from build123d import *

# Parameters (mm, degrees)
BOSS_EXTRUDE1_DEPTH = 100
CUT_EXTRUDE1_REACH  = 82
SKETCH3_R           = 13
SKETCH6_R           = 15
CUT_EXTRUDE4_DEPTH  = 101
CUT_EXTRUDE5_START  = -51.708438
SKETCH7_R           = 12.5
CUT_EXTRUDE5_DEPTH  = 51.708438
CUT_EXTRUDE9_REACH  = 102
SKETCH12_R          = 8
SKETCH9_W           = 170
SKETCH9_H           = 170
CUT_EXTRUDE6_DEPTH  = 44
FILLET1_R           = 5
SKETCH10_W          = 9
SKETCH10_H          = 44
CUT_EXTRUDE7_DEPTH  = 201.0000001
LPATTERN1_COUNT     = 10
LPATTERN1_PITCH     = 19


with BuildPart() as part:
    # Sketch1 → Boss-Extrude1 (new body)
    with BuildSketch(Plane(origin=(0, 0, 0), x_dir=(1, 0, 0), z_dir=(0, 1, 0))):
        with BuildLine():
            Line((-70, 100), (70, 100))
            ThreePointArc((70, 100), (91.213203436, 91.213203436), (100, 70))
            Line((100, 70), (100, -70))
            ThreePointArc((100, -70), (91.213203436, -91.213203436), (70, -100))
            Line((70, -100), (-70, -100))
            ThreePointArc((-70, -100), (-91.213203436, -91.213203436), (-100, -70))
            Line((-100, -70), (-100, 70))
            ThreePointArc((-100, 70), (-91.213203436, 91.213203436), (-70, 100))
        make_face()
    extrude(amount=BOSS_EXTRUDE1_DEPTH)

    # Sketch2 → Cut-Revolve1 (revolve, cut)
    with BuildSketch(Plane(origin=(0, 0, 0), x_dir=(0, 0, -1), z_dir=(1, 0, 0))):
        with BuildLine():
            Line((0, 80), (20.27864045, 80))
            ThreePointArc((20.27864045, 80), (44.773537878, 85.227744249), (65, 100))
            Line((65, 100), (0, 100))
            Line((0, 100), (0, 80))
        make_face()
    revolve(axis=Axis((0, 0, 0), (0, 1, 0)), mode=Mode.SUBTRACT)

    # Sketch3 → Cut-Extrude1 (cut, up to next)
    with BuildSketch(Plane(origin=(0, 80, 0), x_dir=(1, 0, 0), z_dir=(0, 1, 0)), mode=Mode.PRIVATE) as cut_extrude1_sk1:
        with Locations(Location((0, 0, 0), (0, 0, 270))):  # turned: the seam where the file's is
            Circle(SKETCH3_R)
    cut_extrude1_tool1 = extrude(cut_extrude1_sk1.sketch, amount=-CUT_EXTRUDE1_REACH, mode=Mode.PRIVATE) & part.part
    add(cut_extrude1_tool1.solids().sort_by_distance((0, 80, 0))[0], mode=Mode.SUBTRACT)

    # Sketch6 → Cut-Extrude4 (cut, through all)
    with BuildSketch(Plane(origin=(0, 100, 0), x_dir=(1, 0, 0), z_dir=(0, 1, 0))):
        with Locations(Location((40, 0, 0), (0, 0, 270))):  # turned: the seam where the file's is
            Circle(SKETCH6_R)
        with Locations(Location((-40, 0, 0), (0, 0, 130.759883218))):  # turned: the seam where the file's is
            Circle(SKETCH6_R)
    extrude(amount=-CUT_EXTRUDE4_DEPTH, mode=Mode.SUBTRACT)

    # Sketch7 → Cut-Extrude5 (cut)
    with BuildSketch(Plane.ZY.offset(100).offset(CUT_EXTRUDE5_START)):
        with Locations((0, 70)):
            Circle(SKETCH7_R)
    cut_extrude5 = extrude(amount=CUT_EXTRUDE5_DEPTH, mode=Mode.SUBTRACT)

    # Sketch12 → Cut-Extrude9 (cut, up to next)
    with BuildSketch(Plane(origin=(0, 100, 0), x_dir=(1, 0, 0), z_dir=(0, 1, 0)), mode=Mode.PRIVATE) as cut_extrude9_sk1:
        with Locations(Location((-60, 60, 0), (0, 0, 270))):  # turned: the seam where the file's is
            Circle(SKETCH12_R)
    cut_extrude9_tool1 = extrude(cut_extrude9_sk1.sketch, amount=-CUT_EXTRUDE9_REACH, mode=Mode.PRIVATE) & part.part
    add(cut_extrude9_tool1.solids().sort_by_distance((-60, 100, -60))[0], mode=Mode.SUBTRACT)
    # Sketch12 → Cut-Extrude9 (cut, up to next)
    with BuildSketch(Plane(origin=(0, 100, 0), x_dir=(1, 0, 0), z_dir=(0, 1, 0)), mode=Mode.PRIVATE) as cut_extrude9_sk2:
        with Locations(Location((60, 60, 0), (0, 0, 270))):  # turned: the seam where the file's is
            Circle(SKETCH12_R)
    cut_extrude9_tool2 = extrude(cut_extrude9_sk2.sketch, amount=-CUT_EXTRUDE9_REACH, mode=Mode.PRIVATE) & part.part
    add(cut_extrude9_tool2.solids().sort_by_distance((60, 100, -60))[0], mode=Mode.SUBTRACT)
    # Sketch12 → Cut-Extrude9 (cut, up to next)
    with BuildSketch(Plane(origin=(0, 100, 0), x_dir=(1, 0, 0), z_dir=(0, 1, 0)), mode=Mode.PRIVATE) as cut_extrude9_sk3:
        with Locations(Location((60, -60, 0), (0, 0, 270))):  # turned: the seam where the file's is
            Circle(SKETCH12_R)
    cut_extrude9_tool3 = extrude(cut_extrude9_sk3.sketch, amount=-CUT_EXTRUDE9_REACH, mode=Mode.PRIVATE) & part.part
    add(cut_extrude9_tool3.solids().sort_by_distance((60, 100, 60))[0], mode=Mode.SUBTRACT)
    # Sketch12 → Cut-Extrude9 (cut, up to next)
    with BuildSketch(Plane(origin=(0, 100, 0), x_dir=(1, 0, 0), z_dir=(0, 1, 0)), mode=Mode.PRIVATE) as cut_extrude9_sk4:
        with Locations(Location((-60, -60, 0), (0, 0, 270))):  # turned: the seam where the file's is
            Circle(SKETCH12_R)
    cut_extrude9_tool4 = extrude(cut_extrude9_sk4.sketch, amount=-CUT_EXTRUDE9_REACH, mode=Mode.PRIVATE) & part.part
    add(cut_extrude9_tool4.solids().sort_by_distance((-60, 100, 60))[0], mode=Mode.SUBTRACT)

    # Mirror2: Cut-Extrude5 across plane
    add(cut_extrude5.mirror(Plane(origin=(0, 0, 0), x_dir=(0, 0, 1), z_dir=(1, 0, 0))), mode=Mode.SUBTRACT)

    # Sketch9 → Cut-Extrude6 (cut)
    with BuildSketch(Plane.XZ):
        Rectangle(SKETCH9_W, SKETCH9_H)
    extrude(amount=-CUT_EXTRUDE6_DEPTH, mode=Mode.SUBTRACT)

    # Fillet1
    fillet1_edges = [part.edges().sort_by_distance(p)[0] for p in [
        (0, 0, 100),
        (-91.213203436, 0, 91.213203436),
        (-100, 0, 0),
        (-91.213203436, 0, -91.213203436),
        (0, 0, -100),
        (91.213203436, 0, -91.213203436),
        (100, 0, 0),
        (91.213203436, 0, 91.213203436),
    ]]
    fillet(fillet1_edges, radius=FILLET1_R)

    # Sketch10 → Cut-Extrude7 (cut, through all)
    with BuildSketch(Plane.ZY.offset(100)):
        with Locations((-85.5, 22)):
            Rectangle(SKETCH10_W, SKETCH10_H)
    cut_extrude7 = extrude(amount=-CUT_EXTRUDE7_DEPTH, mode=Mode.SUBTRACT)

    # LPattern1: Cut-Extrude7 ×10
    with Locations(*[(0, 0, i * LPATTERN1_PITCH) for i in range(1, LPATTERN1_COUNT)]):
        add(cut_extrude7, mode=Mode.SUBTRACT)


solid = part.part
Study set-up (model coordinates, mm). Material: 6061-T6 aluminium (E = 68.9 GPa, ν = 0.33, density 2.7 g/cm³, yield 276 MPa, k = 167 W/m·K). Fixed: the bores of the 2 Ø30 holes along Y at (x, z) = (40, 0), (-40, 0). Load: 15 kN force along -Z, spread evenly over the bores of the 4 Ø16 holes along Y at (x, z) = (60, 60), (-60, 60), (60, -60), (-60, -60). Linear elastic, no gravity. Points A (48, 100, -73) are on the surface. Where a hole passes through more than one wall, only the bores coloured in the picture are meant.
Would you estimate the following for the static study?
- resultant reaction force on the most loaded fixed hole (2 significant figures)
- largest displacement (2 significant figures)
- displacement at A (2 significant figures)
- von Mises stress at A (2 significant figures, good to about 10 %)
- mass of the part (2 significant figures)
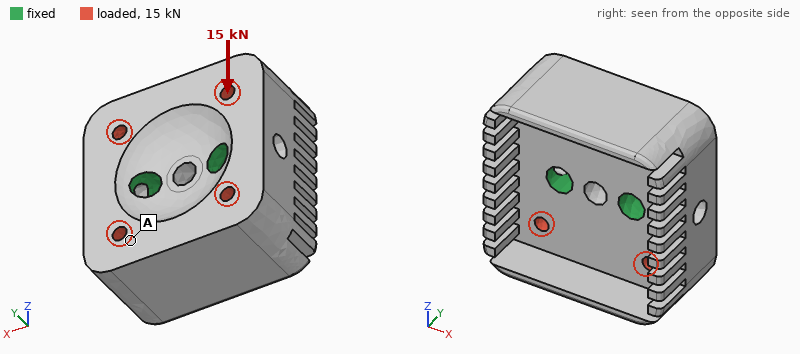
7.5 kN
2.8 µm
2.3 µm
1.0 MPa
5.7 kg
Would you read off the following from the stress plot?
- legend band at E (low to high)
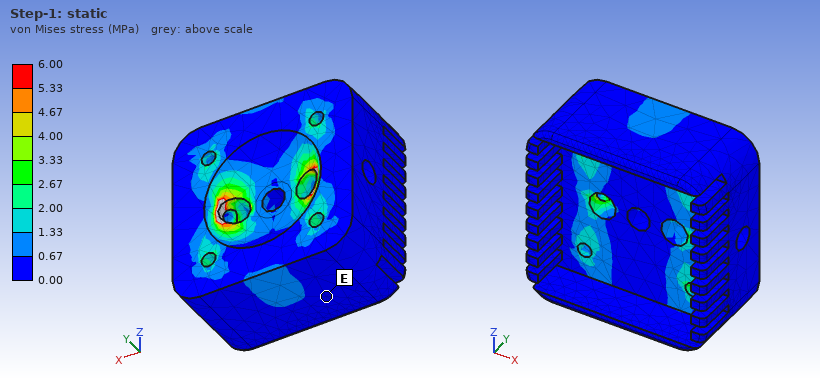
0.00 to 0.67 MPa
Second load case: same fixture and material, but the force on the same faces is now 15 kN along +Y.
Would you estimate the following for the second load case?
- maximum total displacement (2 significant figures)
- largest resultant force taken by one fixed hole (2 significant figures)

10 µm
7.5 kN
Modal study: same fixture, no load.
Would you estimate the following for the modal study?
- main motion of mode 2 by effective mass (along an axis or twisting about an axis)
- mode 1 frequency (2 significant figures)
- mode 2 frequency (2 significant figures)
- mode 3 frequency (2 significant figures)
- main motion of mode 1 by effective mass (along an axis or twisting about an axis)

along Y
2300 Hz
2800 Hz
3100 Hz
twisting about X
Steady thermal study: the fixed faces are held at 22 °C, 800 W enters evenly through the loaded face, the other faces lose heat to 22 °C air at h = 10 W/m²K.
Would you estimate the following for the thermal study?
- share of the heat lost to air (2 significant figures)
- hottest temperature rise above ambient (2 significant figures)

3.5 %
22 K
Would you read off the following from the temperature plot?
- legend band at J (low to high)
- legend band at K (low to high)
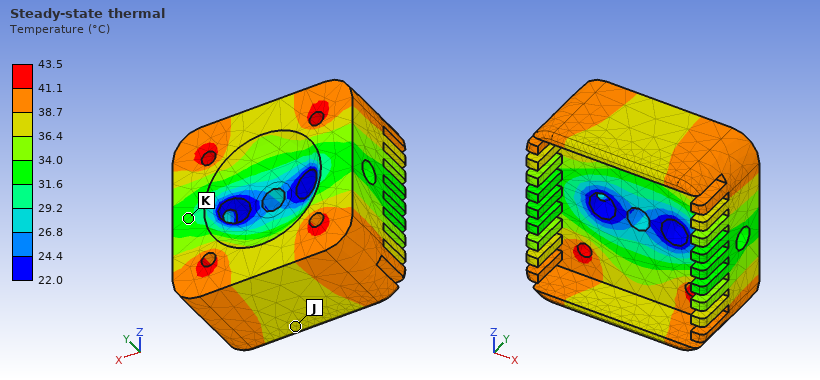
36.4 to 38.7 °C
31.6 to 34.0 °C
